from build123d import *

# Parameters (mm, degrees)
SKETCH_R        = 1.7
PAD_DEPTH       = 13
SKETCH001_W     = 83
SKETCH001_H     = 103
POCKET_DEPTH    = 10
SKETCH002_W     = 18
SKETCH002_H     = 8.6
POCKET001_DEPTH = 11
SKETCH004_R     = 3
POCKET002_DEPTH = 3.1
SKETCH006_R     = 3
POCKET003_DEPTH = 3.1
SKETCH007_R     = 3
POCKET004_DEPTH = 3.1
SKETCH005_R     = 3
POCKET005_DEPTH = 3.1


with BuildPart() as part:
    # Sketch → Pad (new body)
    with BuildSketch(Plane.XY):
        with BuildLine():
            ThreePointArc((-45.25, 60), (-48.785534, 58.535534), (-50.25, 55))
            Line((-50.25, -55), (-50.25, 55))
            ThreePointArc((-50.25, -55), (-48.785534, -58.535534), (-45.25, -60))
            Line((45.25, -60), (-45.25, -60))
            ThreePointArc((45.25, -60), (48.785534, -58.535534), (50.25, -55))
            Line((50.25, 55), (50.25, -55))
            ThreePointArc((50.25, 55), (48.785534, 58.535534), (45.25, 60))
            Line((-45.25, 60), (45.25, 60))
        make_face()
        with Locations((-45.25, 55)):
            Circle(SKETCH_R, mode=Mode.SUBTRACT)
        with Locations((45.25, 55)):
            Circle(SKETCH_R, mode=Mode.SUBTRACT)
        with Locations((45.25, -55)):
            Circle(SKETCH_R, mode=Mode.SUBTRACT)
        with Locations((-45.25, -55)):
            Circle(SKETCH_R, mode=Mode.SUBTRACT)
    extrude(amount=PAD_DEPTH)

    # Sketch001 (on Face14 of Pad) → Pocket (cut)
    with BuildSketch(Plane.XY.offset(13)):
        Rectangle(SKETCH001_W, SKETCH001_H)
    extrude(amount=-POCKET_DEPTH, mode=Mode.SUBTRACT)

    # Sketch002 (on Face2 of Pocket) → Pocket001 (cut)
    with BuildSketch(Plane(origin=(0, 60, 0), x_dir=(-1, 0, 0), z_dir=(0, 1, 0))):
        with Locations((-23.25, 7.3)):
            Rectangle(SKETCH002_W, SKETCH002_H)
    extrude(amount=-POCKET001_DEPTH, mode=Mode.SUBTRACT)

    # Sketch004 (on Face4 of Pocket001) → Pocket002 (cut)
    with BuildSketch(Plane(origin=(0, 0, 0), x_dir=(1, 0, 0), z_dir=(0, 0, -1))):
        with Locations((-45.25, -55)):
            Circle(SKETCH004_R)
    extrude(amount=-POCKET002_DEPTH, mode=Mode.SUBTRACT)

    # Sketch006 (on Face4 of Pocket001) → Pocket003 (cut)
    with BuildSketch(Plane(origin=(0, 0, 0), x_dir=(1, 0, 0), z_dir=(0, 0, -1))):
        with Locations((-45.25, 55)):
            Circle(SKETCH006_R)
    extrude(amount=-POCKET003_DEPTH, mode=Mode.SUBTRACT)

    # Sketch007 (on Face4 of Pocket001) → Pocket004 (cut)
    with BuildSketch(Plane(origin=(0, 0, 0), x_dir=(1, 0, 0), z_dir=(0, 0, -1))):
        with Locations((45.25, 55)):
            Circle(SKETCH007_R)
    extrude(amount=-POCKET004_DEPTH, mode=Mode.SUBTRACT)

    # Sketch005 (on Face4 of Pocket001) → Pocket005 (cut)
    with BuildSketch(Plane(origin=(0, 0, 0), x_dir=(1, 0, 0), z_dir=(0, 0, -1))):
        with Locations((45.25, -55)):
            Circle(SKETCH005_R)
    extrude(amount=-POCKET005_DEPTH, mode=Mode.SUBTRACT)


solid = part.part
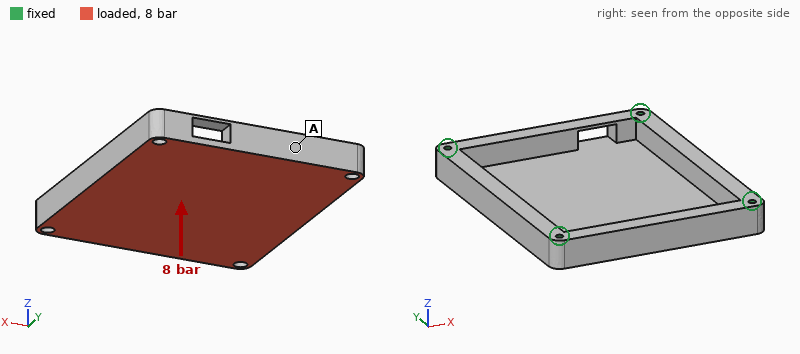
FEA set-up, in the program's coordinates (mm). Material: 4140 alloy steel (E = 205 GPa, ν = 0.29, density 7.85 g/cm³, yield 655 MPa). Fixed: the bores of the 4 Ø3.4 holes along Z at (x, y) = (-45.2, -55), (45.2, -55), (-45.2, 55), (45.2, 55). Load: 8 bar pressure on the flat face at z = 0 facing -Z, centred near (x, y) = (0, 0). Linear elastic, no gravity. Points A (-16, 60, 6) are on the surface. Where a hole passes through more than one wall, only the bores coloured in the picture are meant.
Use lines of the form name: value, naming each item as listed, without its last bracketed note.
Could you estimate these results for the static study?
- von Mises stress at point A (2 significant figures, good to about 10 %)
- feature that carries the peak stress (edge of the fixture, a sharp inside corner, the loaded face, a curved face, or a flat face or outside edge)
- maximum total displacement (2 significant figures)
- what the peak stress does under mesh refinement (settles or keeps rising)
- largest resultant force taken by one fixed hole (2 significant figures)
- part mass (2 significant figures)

von Mises stress at point A: 33 MPa
feature that carries the peak stress: edge of the fixture
maximum total displacement: 0.25 mm
what the peak stress does under mesh refinement: keeps rising
largest resultant force taken by one fixed hole: 4.0 kN
part mass: 540 g
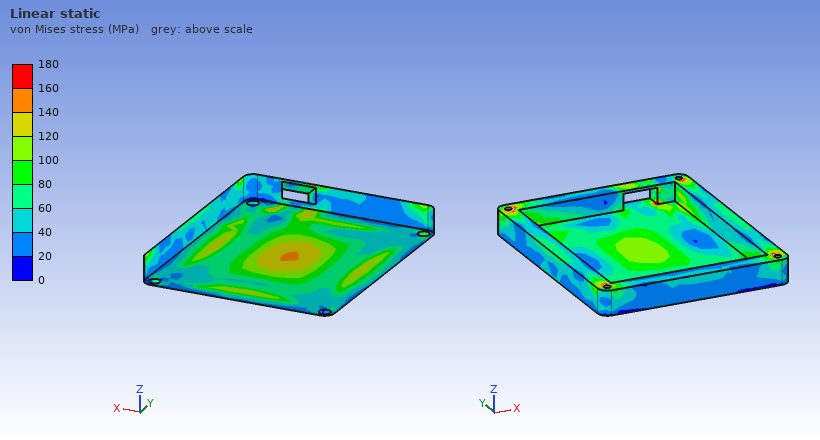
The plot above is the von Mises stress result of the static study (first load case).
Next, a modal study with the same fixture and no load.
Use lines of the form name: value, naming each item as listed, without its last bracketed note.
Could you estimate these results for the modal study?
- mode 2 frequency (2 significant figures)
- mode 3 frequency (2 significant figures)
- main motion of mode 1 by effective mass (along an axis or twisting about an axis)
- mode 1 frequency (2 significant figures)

mode 2 frequency: 4000 Hz
mode 3 frequency: 4100 Hz
main motion of mode 1 by effective mass: along Z
mode 1 frequency: 2300 Hz
